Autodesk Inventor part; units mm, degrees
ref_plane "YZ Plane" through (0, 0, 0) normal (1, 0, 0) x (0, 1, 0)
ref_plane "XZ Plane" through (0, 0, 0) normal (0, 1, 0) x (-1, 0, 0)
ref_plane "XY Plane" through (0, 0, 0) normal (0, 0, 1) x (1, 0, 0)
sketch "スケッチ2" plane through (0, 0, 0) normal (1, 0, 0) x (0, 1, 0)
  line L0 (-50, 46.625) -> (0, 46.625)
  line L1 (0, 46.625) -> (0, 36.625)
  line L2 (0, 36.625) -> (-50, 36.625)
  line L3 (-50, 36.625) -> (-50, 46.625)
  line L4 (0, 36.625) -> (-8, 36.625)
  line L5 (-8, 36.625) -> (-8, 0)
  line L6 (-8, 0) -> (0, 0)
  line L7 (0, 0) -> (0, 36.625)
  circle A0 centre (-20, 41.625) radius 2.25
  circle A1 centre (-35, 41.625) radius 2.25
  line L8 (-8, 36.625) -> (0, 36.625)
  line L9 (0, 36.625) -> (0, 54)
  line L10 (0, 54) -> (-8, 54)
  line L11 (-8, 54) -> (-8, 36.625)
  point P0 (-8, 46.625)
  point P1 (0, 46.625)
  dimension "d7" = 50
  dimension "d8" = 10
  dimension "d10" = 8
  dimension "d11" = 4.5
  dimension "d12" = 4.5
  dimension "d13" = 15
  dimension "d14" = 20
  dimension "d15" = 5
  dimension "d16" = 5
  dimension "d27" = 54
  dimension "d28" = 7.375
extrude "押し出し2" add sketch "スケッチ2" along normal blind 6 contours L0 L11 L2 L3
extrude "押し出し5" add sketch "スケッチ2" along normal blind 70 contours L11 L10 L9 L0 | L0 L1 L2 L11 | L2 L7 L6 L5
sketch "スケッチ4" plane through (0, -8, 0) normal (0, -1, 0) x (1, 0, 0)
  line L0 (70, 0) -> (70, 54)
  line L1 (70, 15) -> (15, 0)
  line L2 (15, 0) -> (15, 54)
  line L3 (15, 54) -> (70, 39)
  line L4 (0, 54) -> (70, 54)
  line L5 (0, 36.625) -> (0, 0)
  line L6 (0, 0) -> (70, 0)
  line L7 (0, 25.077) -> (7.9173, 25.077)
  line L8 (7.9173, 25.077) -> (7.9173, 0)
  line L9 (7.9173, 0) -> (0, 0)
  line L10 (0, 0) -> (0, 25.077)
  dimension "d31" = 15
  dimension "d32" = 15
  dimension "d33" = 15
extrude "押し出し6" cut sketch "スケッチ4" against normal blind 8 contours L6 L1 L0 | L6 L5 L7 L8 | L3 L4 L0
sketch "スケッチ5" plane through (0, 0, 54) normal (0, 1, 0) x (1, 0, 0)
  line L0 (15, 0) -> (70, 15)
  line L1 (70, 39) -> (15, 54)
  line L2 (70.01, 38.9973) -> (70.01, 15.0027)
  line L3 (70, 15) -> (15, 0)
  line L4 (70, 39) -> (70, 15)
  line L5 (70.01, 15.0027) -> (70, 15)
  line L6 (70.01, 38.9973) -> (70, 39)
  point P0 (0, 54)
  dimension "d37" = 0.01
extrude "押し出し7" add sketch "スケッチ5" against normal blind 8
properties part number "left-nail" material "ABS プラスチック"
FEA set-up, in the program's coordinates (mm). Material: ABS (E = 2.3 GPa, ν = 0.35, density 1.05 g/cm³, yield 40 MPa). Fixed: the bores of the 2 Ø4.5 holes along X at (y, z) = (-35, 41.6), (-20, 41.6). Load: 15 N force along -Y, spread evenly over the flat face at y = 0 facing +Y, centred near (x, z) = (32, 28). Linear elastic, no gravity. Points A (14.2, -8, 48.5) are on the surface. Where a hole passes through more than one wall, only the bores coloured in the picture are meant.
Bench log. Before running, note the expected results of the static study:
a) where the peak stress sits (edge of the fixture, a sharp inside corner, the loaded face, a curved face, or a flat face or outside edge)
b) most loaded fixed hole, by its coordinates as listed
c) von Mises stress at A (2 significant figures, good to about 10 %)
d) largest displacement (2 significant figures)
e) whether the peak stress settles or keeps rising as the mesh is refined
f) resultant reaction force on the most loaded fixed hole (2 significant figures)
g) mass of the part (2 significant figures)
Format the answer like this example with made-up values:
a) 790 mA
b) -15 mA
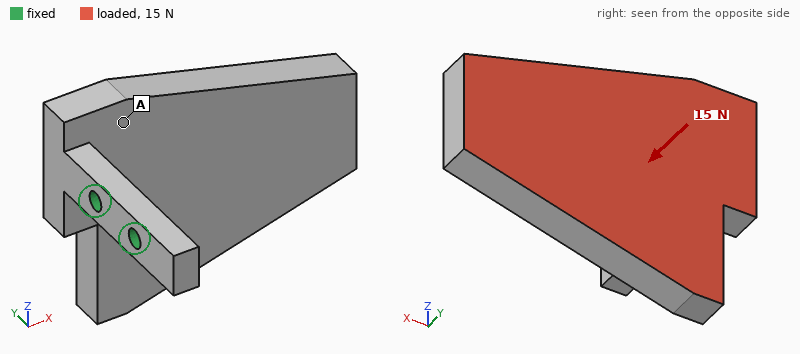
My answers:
a) edge of the fixture
b) (-20, 41.6)
c) 1.00 MPa
d) 1.2 mm
e) keeps rising
f) 15 N
g) 26 g
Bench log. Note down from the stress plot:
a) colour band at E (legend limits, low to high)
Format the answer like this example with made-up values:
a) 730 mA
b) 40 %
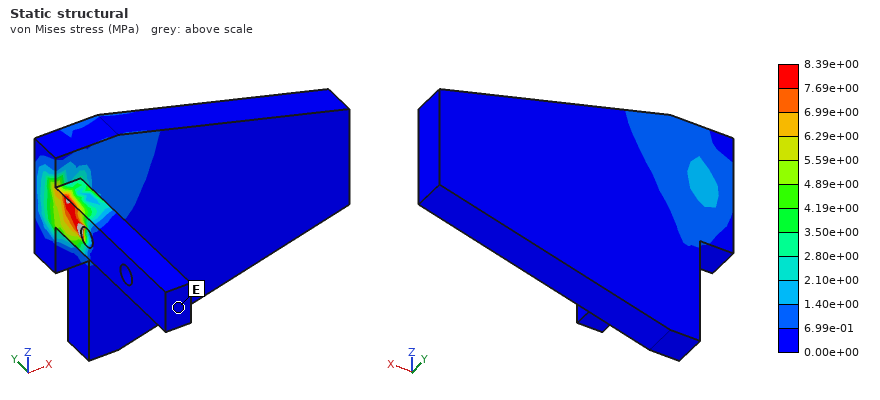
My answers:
a) 0.00e+00 to 6.99e-01 MPa
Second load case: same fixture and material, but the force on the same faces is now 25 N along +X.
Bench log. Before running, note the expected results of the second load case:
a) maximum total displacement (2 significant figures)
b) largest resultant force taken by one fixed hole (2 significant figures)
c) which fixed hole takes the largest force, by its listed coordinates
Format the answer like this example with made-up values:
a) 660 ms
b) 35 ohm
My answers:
a) 1.1 mm
b) 27 N
c) (-20, 41.6)
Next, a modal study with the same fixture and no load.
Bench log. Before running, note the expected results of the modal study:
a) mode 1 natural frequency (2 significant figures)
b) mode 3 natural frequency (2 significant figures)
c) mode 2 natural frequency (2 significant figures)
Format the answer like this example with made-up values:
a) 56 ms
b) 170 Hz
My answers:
a) 150 Hz
b) 520 Hz
c) 160 Hz
